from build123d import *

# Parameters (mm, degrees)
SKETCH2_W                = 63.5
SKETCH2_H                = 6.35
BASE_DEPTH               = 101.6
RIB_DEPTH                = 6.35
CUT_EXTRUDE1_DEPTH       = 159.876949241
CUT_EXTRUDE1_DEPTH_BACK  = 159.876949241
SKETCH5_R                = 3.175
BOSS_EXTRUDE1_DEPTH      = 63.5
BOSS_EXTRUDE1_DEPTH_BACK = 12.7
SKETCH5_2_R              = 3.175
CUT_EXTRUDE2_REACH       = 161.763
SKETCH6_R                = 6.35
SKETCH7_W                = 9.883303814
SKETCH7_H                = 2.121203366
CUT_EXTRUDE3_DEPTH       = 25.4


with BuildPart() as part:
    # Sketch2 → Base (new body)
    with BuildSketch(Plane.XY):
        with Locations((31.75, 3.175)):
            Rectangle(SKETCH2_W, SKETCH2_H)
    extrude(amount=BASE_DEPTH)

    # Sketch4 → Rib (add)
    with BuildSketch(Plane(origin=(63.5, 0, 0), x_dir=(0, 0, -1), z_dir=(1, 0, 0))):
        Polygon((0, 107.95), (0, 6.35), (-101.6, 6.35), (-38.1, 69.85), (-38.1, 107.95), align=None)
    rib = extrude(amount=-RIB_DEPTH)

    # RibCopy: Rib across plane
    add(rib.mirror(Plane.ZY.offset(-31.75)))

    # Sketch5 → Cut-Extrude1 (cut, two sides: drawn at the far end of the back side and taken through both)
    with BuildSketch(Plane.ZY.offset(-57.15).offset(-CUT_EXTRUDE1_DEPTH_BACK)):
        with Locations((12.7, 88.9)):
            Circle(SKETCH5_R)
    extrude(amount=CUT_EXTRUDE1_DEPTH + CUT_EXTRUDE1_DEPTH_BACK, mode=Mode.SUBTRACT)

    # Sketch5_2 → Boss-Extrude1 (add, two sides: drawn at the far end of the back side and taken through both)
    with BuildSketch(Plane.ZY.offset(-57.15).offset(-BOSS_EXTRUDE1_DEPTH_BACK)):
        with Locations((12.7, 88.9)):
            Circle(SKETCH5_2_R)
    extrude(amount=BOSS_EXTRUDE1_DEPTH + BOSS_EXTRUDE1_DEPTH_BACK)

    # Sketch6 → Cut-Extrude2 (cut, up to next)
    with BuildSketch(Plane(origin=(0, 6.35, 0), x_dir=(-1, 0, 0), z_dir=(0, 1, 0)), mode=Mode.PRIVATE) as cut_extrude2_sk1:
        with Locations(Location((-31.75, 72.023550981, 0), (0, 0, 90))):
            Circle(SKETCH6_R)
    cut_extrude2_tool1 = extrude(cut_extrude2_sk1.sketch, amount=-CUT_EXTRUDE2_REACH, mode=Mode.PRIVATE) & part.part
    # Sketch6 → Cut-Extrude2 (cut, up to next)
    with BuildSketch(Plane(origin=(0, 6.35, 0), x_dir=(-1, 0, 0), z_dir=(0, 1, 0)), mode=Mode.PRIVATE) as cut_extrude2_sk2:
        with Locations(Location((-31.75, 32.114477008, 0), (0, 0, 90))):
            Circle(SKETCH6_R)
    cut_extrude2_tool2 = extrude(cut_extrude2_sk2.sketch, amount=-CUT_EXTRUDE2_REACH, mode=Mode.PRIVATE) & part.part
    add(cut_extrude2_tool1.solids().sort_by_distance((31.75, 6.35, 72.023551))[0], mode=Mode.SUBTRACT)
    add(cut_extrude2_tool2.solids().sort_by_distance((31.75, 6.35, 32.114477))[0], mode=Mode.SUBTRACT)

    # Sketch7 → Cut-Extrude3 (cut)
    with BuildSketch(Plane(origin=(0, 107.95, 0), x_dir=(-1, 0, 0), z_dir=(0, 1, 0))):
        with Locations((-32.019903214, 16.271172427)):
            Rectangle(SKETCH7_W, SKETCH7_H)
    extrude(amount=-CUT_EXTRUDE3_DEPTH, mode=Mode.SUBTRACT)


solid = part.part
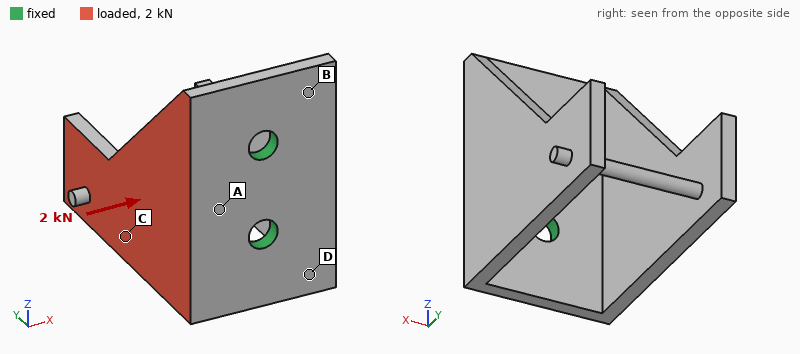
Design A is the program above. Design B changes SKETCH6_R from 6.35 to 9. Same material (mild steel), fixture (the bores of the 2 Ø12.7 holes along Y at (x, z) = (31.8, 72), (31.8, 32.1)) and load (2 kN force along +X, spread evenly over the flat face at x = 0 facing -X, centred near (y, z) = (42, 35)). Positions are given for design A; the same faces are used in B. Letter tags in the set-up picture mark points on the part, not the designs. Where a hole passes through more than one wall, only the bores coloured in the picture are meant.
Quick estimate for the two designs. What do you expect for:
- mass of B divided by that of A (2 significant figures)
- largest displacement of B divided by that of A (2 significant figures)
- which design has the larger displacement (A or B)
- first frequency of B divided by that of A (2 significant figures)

0.99
0.92
A
1.0
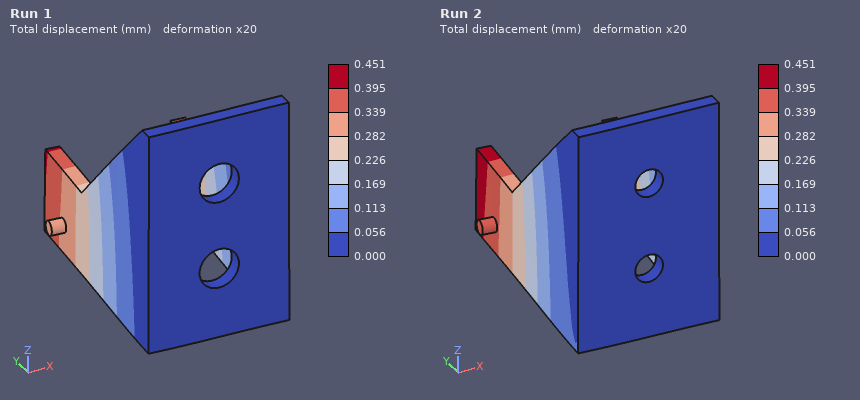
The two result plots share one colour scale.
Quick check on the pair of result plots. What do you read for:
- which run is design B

Run 1
